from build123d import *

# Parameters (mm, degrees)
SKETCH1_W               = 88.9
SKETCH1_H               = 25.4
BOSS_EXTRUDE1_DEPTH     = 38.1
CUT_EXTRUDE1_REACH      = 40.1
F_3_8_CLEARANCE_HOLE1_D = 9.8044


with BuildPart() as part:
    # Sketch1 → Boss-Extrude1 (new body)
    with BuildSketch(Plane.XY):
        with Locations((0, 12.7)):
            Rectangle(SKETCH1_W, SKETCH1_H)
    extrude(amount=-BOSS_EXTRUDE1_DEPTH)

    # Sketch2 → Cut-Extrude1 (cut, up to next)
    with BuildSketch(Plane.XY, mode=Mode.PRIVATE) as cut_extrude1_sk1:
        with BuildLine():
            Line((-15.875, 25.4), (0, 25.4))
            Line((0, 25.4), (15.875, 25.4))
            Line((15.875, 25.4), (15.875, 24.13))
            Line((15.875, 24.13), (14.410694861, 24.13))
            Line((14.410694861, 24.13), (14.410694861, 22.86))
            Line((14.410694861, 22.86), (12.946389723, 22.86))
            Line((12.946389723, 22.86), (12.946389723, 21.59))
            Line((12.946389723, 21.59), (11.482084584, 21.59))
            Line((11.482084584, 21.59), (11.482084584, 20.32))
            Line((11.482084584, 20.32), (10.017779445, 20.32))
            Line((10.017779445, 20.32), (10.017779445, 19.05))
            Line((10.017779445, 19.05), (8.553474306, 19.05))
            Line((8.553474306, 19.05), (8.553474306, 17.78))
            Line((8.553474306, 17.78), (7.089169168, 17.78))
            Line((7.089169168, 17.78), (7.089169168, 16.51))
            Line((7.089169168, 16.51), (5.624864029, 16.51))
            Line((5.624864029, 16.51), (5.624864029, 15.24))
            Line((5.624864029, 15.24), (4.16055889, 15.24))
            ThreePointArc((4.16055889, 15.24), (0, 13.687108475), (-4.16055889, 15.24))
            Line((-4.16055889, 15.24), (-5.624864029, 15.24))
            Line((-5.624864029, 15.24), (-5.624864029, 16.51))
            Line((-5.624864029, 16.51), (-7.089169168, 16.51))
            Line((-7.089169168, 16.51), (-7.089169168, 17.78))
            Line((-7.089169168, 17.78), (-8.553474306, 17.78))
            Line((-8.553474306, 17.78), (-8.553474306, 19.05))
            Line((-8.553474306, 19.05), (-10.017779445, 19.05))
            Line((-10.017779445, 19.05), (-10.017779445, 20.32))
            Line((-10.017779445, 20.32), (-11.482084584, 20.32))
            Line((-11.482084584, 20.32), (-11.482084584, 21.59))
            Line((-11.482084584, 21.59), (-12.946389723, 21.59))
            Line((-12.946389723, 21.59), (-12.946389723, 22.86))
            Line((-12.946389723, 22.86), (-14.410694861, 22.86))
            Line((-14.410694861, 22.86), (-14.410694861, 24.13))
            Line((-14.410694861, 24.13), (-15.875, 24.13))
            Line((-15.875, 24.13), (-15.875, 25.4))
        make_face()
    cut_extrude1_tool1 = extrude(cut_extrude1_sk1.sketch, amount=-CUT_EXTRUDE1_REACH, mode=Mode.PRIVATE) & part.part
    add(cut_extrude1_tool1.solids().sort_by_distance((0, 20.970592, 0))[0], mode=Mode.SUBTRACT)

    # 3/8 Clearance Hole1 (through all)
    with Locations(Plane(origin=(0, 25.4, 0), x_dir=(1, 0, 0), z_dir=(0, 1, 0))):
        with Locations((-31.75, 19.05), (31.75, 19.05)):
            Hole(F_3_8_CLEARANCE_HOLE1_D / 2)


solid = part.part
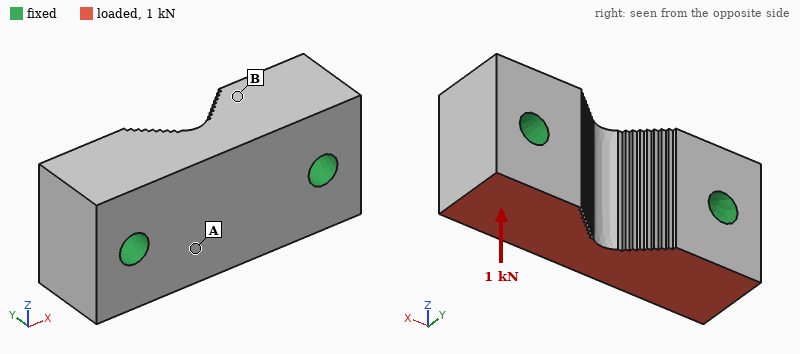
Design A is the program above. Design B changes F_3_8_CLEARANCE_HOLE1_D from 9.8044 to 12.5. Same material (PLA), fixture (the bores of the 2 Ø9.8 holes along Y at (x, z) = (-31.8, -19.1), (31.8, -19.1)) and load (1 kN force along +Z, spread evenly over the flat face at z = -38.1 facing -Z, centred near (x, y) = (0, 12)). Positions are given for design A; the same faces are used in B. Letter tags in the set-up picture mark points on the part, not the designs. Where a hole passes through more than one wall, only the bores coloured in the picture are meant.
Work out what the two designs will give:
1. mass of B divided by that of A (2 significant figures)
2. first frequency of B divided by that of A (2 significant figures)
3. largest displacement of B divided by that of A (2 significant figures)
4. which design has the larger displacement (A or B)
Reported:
0.97
1.1
0.87
A
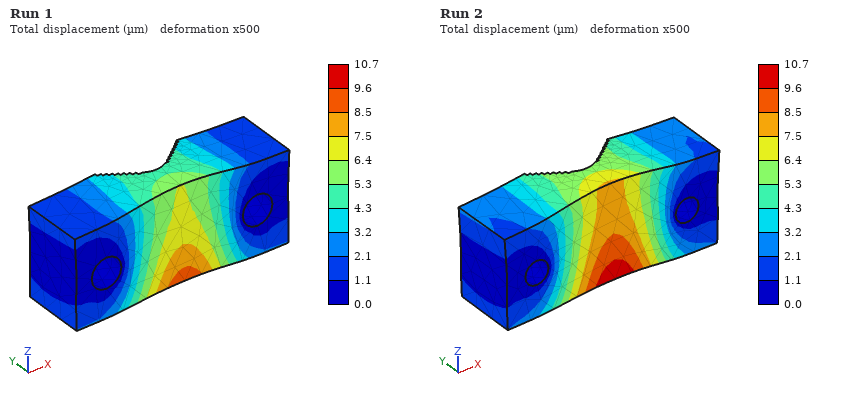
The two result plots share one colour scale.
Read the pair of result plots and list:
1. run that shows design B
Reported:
Run 1
